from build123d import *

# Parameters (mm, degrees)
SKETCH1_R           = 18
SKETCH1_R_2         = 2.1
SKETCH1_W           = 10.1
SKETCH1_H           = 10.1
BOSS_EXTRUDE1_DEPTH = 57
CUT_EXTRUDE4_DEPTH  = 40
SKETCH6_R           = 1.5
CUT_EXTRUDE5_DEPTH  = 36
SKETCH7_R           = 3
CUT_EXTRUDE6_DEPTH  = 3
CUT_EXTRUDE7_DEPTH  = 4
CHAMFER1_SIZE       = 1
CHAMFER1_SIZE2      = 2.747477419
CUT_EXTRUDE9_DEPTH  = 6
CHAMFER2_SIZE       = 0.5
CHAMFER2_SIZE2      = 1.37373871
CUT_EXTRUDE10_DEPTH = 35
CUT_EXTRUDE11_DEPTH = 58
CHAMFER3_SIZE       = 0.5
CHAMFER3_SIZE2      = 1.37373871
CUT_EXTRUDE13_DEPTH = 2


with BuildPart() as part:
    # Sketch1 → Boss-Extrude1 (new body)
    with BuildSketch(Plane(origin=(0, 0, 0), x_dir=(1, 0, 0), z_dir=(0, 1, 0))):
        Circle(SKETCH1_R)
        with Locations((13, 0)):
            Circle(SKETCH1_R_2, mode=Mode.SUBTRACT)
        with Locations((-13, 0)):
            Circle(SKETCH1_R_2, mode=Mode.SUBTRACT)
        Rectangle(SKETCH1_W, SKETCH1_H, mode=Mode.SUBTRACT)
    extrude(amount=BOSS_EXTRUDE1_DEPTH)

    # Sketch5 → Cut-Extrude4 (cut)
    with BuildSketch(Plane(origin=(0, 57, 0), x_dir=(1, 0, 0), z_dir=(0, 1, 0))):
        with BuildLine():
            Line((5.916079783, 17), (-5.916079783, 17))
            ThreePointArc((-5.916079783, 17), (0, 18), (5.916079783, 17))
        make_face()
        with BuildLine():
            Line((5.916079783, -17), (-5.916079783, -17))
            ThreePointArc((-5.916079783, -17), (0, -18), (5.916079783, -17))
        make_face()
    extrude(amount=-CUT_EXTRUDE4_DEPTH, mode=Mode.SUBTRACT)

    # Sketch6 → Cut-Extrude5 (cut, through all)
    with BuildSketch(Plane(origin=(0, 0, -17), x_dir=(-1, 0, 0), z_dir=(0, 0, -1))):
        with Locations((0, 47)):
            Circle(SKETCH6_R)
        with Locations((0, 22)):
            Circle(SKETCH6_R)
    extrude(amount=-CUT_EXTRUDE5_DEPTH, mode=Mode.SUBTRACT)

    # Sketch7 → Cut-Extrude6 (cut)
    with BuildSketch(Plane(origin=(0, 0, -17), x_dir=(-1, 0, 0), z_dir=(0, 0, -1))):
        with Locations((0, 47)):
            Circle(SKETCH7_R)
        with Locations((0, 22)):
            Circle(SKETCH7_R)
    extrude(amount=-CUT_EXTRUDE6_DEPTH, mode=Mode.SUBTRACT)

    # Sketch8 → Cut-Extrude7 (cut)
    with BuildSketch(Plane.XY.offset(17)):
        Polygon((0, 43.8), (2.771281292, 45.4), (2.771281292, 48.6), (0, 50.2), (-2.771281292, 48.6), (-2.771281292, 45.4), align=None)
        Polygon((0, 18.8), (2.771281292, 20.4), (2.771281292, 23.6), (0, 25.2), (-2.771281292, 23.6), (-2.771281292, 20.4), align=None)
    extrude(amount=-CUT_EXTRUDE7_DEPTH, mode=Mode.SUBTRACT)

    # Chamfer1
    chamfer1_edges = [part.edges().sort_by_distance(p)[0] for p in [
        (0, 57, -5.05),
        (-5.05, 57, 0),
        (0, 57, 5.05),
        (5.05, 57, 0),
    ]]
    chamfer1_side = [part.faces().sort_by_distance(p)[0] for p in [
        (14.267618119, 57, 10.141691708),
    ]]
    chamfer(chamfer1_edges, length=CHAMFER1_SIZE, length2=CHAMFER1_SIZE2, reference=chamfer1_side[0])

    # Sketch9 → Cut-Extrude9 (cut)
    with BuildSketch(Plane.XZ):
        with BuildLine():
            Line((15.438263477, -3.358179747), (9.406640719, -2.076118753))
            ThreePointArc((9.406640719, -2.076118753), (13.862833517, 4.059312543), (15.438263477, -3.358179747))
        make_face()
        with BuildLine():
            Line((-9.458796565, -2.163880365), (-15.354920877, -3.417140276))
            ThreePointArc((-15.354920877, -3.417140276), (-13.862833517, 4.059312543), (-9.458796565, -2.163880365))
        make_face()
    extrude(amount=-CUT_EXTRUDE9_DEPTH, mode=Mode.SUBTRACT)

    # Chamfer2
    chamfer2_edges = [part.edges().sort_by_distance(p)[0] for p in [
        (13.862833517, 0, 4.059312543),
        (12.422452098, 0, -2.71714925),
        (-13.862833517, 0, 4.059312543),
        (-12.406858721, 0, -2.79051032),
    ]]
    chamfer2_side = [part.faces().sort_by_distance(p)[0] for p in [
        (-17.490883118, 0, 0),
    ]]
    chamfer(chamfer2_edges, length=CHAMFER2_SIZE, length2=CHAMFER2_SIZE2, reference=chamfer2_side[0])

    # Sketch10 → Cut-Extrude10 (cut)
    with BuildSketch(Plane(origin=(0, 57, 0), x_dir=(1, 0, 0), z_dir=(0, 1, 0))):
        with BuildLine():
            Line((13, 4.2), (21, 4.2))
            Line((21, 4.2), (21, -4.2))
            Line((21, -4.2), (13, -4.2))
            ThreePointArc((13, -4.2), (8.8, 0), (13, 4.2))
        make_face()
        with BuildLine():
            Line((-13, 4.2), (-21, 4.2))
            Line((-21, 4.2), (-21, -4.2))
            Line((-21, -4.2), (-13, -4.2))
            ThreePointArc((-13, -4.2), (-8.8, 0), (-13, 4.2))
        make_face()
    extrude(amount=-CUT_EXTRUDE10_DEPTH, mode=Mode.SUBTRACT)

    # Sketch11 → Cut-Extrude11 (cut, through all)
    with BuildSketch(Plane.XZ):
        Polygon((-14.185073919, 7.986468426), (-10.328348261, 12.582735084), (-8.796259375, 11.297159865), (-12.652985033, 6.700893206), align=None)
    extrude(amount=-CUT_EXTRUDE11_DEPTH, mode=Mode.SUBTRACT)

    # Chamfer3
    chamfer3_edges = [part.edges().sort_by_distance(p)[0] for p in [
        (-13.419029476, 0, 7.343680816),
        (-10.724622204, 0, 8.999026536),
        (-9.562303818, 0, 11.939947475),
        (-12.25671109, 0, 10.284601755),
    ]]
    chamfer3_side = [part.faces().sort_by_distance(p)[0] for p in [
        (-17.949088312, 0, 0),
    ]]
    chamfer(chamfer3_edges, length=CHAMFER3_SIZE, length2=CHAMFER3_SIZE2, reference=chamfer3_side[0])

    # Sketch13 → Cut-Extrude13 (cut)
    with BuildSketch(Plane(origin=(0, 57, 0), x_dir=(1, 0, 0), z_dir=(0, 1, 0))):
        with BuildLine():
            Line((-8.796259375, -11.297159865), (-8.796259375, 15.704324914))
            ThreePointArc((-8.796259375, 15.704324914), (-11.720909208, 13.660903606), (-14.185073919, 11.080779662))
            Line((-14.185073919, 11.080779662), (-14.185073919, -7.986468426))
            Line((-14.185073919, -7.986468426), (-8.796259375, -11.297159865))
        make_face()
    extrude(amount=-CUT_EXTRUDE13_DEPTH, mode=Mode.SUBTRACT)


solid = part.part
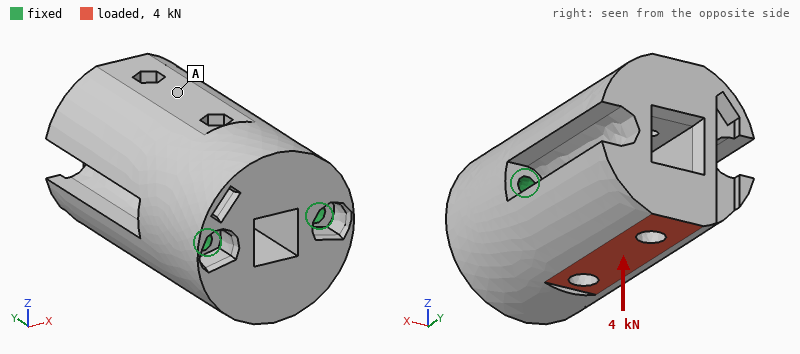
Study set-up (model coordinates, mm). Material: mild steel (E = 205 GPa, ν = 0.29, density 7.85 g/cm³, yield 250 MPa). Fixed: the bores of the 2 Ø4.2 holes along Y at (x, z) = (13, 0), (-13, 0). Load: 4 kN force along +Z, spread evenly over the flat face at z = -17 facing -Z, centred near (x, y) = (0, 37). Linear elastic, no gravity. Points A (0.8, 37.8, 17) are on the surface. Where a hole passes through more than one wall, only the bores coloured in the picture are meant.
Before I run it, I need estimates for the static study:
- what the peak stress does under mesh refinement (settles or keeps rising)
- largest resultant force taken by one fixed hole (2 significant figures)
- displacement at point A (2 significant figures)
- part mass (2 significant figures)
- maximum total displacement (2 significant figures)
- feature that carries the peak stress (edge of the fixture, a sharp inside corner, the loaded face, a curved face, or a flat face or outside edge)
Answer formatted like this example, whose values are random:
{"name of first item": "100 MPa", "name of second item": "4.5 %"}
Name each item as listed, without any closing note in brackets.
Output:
{"what the peak stress does under mesh refinement": "keeps rising", "largest resultant force taken by one fixed hole": "2.0 kN", "displacement at point A": "10 µm", "part mass": "350 g", "maximum total displacement": "18 µm", "feature that carries the peak stress": "edge of the fixture"}
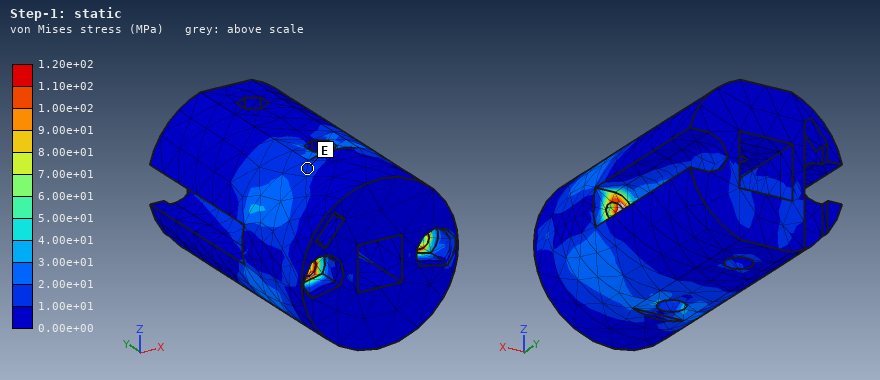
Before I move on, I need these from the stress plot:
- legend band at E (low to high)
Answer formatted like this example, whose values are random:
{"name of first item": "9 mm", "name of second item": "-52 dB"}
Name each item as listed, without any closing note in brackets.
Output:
{"legend band at E": "1.00e+01 to 2.00e+01 MPa"}
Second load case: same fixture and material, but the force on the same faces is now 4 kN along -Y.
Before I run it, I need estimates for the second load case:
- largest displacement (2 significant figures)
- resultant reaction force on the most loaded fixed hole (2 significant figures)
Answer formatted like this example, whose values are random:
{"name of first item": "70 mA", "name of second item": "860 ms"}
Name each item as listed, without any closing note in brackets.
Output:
{"largest displacement": "14 µm", "resultant reaction force on the most loaded fixed hole": "2.0 kN"}
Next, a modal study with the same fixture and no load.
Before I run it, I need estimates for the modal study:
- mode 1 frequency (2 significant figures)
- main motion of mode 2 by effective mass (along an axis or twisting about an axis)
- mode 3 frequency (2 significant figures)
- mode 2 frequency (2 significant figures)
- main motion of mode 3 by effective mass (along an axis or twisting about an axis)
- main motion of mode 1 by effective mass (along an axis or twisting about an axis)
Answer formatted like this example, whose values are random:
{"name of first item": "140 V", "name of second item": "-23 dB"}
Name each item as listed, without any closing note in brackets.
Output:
{"mode 1 frequency": "6100 Hz", "main motion of mode 2 by effective mass": "along X", "mode 3 frequency": "15 kHz", "mode 2 frequency": "9500 Hz", "main motion of mode 3 by effective mass": "twisting about Y", "main motion of mode 1 by effective mass": "along Z"}
